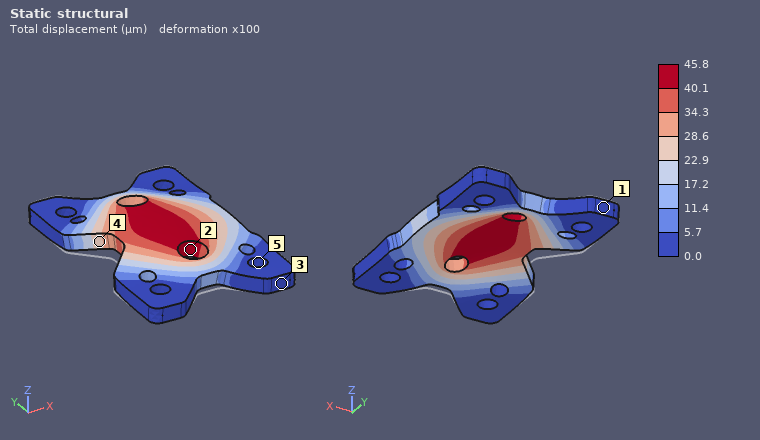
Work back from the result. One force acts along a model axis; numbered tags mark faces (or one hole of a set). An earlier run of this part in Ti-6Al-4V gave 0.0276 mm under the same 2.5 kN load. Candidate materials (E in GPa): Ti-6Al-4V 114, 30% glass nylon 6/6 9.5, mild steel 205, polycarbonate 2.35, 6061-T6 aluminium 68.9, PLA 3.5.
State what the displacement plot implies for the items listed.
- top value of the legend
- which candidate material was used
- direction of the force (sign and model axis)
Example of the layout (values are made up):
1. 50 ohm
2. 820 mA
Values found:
1. 45.8 µm
2. 6061-T6 aluminium
3. +Z
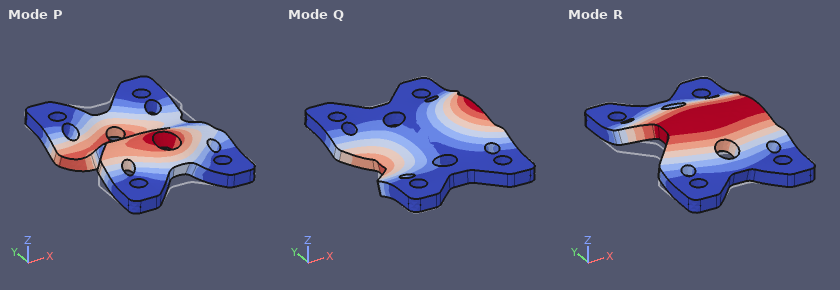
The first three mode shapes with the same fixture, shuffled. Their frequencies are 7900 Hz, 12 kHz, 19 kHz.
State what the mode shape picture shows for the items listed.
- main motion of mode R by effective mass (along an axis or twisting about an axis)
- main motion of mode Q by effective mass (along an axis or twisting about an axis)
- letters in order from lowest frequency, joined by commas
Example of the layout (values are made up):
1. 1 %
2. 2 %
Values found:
1. along Z
2. twisting about Y
3. R, Q, P
